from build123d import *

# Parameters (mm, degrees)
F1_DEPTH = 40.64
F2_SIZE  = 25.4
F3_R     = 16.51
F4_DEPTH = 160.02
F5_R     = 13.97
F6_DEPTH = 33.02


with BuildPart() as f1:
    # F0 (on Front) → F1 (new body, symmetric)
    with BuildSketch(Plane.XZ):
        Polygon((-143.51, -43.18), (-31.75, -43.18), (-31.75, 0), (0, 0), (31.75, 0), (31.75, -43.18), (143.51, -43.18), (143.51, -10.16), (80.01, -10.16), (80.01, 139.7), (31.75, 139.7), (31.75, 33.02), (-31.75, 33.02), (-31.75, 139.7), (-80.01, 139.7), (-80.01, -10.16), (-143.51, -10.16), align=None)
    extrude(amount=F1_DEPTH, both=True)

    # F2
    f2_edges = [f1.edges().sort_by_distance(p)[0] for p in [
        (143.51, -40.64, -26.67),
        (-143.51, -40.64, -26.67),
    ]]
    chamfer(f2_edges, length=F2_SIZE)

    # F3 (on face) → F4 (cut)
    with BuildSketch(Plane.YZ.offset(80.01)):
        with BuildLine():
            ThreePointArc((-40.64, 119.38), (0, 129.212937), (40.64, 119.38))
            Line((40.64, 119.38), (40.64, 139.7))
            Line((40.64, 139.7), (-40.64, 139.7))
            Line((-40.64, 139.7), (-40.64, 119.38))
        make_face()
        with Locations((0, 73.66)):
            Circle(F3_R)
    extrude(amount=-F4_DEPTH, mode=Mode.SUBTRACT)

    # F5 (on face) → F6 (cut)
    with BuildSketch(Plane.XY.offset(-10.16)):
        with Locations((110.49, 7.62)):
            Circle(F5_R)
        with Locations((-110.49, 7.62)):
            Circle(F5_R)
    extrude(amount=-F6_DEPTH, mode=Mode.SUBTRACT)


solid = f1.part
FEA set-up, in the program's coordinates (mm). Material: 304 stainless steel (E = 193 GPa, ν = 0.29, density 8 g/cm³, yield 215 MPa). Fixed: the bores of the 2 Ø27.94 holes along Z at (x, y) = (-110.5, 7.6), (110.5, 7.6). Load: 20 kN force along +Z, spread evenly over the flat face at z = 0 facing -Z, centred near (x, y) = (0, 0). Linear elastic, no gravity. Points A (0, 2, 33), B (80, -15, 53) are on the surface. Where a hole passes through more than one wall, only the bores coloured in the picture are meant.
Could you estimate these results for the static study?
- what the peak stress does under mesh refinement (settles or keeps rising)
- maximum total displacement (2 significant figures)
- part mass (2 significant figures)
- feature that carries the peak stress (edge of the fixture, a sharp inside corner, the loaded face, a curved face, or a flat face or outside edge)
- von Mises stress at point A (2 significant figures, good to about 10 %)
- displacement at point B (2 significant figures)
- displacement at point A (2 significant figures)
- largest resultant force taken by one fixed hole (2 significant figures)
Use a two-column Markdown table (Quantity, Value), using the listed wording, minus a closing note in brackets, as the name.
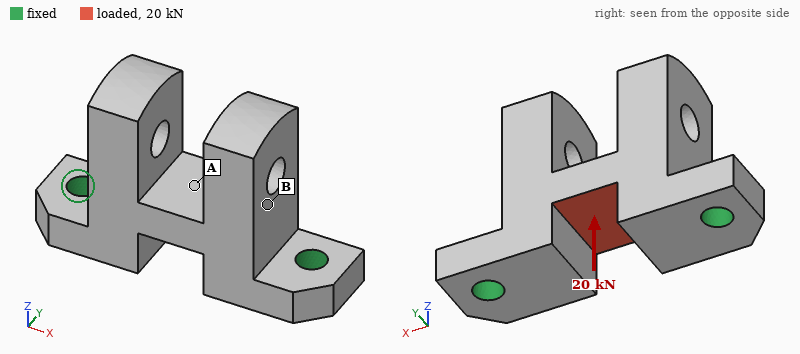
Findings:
| Quantity | Value |
|---|---|
| what the peak stress does under mesh refinement | keeps rising |
| maximum total displacement | 13 µm |
| part mass | 14 kg |
| feature that carries the peak stress | edge of the fixture |
| von Mises stress at point A | 14 MPa |
| displacement at point B | 5.9 µm |
| displacement at point A | 9.1 µm |
| largest resultant force taken by one fixed hole | 15 kN |
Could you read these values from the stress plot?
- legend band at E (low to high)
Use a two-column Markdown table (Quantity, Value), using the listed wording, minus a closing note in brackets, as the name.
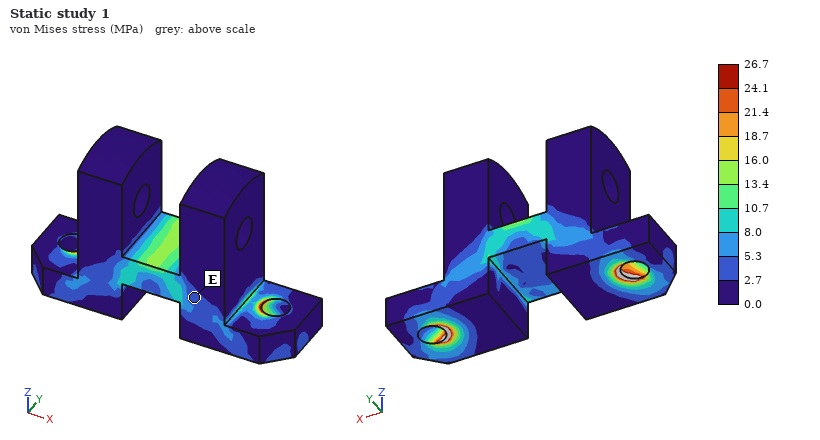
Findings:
| Quantity | Value |
|---|---|
| legend band at E | 2.7 to 5.3 MPa |
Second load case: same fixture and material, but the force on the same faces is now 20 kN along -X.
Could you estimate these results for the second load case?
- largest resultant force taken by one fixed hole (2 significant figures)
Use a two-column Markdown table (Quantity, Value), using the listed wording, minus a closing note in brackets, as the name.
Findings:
| Quantity | Value |
|---|---|
| largest resultant force taken by one fixed hole | 10 kN |
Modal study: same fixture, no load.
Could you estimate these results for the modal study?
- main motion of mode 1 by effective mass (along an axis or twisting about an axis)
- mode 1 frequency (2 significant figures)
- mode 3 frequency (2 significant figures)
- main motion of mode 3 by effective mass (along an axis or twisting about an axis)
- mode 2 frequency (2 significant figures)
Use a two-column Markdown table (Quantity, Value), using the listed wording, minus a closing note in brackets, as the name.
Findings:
| Quantity | Value |
|---|---|
| main motion of mode 1 by effective mass | along Y |
| mode 1 frequency | 980 Hz |
| mode 3 frequency | 1900 Hz |
| main motion of mode 3 by effective mass | along X |
| mode 2 frequency | 1700 Hz |
